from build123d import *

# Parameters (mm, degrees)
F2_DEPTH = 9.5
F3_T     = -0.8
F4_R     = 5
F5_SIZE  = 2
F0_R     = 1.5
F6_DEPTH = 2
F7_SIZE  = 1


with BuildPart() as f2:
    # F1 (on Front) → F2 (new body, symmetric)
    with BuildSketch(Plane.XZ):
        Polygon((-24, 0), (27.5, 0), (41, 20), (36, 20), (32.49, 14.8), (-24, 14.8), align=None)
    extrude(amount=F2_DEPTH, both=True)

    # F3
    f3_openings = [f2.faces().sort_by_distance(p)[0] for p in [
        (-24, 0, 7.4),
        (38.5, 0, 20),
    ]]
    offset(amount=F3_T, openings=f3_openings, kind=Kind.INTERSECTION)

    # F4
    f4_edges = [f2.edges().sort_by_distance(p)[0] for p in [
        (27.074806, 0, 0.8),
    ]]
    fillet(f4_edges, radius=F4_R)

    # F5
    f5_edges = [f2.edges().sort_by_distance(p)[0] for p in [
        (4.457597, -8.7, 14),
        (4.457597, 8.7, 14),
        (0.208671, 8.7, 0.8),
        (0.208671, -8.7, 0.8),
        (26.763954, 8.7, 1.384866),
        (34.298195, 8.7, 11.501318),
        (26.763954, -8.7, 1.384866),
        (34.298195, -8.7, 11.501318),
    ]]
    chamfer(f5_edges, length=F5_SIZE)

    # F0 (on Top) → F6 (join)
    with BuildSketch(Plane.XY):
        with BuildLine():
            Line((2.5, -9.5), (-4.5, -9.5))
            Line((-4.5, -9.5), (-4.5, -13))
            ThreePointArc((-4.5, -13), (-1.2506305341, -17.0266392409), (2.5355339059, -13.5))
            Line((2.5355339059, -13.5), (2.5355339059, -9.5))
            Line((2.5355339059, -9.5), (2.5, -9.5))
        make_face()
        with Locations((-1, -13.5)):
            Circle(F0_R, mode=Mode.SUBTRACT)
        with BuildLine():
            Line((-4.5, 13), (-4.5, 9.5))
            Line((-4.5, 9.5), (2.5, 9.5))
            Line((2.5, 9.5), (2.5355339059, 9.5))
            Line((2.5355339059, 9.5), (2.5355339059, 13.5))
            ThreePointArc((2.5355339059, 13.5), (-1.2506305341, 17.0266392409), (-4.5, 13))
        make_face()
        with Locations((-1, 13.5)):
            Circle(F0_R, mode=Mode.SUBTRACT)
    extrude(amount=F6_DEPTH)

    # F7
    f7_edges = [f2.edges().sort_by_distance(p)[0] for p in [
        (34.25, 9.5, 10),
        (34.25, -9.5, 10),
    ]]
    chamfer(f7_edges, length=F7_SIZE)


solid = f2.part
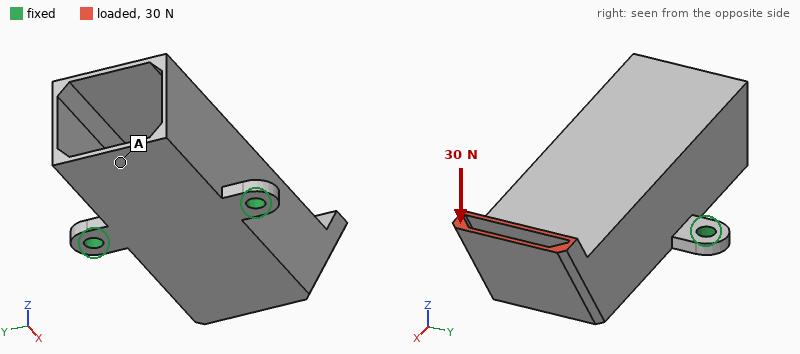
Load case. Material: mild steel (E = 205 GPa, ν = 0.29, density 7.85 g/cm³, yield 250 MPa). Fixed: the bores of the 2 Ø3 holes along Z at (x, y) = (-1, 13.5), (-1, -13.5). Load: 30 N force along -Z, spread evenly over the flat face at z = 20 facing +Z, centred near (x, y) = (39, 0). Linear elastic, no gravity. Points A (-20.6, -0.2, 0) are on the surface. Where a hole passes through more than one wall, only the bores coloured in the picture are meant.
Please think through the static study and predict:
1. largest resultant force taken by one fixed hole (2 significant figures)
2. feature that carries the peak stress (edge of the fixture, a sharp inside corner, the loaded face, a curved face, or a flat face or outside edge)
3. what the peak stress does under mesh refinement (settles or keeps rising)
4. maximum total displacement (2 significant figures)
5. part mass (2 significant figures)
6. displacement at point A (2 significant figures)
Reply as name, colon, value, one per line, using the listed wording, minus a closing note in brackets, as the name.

largest resultant force taken by one fixed hole: 15 N
feature that carries the peak stress: edge of the fixture
what the peak stress does under mesh refinement: keeps rising
maximum total displacement: 68 µm
part mass: 31 g
displacement at point A: 26 µm
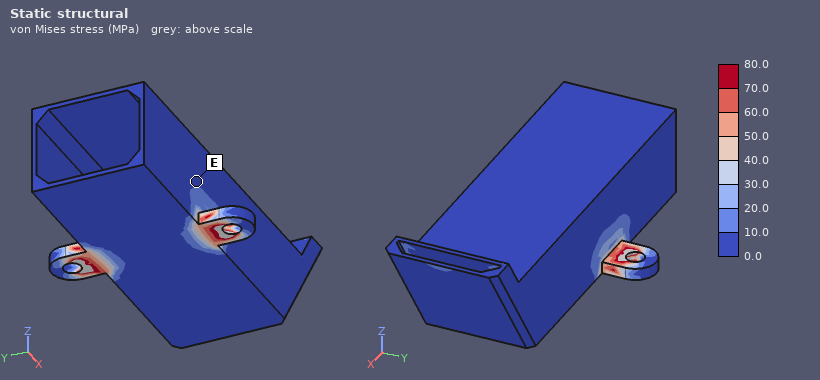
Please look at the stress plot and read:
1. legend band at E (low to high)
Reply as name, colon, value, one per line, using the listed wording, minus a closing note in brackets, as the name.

legend band at E: 0.0 to 10.0 MPa
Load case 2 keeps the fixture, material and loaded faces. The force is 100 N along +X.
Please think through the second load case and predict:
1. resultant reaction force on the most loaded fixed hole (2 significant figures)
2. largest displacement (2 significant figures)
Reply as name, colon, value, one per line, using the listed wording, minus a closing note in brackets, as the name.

resultant reaction force on the most loaded fixed hole: 50 N
largest displacement: 0.12 mm
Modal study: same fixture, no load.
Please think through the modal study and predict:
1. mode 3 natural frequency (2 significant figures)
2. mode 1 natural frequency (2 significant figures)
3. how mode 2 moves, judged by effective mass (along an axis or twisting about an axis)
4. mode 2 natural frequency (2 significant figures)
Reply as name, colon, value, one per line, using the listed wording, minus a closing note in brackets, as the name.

mode 3 natural frequency: 5600 Hz
mode 1 natural frequency: 1200 Hz
how mode 2 moves, judged by effective mass: along Y
mode 2 natural frequency: 3100 Hz
